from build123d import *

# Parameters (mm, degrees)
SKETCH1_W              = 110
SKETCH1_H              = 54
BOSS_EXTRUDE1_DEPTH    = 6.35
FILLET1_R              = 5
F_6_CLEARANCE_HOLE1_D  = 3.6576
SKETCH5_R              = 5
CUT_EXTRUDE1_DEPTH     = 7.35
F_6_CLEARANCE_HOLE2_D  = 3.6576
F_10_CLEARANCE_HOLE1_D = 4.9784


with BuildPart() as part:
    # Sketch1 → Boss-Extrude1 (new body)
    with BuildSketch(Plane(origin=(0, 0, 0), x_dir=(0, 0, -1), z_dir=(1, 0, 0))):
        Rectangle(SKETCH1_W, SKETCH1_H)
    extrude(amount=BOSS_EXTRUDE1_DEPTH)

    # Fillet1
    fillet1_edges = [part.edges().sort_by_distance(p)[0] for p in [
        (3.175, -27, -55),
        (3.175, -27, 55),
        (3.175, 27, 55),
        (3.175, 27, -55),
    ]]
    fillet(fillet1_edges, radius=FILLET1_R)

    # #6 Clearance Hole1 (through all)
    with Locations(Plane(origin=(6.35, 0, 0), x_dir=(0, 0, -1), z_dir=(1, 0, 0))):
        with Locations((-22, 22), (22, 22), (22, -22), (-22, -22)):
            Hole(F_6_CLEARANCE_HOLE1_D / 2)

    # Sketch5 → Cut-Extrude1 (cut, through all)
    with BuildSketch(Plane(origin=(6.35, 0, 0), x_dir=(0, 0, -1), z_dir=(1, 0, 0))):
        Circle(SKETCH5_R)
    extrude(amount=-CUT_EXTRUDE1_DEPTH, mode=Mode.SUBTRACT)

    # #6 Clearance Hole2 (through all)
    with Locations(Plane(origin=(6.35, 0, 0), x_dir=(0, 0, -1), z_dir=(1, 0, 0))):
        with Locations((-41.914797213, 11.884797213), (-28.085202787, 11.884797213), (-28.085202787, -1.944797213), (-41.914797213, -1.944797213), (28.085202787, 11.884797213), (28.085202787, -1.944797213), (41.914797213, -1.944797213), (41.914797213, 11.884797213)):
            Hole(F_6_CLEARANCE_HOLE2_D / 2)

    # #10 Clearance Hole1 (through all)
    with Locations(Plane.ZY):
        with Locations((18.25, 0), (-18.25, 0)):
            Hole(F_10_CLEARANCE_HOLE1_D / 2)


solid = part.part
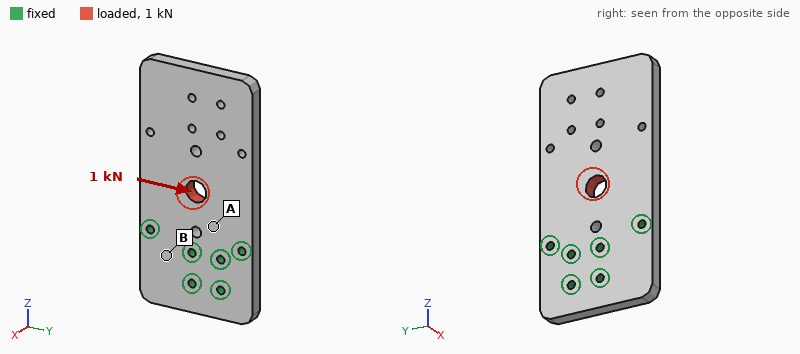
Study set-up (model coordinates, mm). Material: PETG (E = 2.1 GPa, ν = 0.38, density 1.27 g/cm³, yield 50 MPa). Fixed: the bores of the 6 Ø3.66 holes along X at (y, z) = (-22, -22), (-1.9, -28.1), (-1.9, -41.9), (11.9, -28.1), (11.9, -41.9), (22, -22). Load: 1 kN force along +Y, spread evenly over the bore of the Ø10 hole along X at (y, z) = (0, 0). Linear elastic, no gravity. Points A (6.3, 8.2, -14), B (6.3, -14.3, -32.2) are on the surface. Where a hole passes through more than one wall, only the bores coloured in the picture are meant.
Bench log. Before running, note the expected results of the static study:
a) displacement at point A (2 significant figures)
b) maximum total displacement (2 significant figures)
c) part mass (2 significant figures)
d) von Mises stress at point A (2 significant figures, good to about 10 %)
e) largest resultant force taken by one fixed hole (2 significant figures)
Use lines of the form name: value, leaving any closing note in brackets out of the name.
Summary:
displacement at point A: 0.050 mm
maximum total displacement: 0.22 mm
part mass: 46 g
von Mises stress at point A: 5.8 MPa
largest resultant force taken by one fixed hole: 620 N
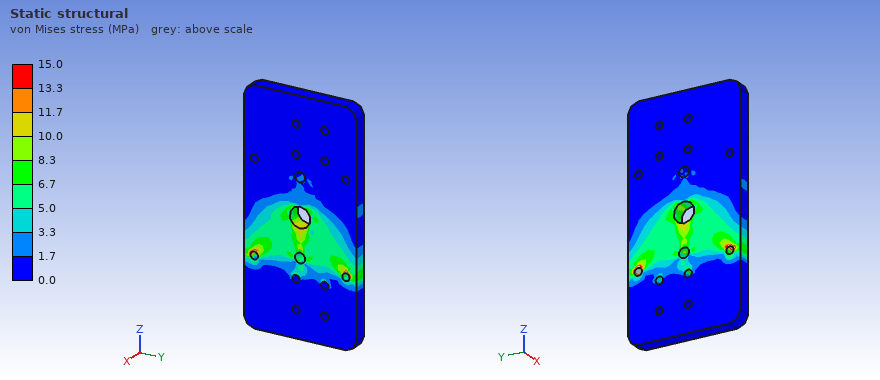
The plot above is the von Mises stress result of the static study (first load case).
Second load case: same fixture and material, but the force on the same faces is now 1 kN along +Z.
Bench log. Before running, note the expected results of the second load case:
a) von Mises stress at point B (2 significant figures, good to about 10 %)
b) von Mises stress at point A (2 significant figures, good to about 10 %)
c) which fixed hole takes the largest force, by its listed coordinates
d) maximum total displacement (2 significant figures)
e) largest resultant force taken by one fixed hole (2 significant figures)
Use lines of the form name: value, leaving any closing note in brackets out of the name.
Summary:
von Mises stress at point B: 0.94 MPa
von Mises stress at point A: 3.8 MPa
which fixed hole takes the largest force, by its listed coordinates: (-22, -22)
maximum total displacement: 69 µm
largest resultant force taken by one fixed hole: 320 N
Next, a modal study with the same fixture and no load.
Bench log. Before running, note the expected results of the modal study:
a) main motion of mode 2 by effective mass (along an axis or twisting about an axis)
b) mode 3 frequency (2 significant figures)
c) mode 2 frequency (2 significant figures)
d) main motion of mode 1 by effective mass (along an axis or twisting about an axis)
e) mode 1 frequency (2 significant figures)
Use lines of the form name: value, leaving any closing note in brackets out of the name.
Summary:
main motion of mode 2 by effective mass: twisting about Z
mode 3 frequency: 1300 Hz
mode 2 frequency: 670 Hz
main motion of mode 1 by effective mass: along X
mode 1 frequency: 210 Hz
